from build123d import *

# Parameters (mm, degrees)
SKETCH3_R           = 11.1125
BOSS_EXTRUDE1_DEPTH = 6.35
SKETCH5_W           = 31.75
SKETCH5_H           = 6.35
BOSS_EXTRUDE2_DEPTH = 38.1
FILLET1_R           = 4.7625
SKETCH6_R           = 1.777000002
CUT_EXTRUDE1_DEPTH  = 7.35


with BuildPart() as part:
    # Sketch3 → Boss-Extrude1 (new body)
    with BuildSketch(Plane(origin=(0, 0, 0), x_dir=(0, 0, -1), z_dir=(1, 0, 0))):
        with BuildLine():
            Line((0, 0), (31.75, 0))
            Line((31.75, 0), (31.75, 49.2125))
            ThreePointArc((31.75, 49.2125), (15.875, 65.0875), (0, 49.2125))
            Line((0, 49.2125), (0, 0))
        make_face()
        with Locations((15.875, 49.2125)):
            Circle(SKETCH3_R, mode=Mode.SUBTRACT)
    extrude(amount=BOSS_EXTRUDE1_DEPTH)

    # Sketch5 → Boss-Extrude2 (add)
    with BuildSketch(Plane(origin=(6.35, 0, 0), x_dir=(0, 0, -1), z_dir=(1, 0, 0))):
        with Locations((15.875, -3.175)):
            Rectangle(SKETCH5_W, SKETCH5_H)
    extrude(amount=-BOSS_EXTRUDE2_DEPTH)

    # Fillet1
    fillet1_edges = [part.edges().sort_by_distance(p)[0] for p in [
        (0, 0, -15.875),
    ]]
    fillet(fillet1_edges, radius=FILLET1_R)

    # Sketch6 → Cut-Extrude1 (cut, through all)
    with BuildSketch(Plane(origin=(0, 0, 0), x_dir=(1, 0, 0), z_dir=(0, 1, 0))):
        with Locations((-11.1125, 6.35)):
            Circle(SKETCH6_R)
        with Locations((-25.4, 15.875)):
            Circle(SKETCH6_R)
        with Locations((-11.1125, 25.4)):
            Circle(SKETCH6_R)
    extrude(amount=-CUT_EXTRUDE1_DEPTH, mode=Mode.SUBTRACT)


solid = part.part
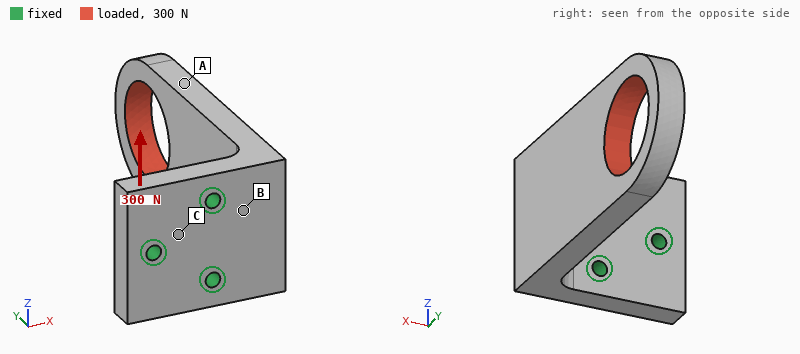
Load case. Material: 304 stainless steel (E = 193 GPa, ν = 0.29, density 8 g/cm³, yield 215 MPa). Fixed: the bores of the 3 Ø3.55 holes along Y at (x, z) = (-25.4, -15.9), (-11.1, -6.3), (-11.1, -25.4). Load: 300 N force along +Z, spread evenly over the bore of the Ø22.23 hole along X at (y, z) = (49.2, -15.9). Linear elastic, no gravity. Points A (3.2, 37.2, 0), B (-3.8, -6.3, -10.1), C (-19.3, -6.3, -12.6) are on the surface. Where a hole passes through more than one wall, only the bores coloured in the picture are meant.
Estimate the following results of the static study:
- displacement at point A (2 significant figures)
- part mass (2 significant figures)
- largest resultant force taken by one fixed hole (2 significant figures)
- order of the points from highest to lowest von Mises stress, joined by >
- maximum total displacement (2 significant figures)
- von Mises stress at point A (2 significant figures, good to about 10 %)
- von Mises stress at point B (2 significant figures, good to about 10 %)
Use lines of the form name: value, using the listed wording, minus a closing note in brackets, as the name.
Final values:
displacement at point A: 22 µm
part mass: 140 g
largest resultant force taken by one fixed hole: 740 N
order of the points from highest to lowest von Mises stress, joined by >: B > A > C
maximum total displacement: 39 µm
von Mises stress at point A: 12 MPa
von Mises stress at point B: 23 MPa
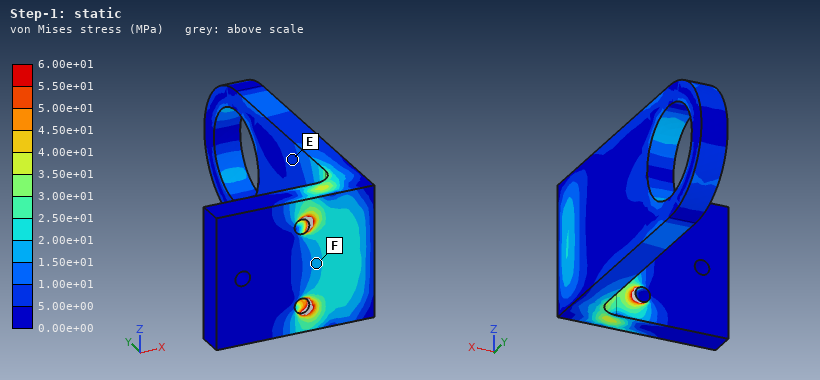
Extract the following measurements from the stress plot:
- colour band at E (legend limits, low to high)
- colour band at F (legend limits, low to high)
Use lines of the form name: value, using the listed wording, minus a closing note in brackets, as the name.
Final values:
colour band at E: 5.00e+00 to 1.00e+01 MPa
colour band at F: 1.50e+01 to 2.00e+01 MPa
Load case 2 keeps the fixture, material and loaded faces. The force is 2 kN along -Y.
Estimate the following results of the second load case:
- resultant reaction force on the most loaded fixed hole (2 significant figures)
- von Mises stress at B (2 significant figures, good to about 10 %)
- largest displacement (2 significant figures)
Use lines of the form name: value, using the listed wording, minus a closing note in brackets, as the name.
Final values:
resultant reaction force on the most loaded fixed hole: 1.2 kN
von Mises stress at B: 56 MPa
largest displacement: 0.11 mm
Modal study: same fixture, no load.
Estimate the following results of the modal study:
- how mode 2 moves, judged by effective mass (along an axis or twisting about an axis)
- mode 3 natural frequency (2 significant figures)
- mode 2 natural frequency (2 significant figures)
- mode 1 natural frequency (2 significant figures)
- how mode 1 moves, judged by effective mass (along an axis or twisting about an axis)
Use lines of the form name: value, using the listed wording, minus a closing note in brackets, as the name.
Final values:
how mode 2 moves, judged by effective mass: along Z
mode 3 natural frequency: 5000 Hz
mode 2 natural frequency: 2800 Hz
mode 1 natural frequency: 1200 Hz
how mode 1 moves, judged by effective mass: along X
